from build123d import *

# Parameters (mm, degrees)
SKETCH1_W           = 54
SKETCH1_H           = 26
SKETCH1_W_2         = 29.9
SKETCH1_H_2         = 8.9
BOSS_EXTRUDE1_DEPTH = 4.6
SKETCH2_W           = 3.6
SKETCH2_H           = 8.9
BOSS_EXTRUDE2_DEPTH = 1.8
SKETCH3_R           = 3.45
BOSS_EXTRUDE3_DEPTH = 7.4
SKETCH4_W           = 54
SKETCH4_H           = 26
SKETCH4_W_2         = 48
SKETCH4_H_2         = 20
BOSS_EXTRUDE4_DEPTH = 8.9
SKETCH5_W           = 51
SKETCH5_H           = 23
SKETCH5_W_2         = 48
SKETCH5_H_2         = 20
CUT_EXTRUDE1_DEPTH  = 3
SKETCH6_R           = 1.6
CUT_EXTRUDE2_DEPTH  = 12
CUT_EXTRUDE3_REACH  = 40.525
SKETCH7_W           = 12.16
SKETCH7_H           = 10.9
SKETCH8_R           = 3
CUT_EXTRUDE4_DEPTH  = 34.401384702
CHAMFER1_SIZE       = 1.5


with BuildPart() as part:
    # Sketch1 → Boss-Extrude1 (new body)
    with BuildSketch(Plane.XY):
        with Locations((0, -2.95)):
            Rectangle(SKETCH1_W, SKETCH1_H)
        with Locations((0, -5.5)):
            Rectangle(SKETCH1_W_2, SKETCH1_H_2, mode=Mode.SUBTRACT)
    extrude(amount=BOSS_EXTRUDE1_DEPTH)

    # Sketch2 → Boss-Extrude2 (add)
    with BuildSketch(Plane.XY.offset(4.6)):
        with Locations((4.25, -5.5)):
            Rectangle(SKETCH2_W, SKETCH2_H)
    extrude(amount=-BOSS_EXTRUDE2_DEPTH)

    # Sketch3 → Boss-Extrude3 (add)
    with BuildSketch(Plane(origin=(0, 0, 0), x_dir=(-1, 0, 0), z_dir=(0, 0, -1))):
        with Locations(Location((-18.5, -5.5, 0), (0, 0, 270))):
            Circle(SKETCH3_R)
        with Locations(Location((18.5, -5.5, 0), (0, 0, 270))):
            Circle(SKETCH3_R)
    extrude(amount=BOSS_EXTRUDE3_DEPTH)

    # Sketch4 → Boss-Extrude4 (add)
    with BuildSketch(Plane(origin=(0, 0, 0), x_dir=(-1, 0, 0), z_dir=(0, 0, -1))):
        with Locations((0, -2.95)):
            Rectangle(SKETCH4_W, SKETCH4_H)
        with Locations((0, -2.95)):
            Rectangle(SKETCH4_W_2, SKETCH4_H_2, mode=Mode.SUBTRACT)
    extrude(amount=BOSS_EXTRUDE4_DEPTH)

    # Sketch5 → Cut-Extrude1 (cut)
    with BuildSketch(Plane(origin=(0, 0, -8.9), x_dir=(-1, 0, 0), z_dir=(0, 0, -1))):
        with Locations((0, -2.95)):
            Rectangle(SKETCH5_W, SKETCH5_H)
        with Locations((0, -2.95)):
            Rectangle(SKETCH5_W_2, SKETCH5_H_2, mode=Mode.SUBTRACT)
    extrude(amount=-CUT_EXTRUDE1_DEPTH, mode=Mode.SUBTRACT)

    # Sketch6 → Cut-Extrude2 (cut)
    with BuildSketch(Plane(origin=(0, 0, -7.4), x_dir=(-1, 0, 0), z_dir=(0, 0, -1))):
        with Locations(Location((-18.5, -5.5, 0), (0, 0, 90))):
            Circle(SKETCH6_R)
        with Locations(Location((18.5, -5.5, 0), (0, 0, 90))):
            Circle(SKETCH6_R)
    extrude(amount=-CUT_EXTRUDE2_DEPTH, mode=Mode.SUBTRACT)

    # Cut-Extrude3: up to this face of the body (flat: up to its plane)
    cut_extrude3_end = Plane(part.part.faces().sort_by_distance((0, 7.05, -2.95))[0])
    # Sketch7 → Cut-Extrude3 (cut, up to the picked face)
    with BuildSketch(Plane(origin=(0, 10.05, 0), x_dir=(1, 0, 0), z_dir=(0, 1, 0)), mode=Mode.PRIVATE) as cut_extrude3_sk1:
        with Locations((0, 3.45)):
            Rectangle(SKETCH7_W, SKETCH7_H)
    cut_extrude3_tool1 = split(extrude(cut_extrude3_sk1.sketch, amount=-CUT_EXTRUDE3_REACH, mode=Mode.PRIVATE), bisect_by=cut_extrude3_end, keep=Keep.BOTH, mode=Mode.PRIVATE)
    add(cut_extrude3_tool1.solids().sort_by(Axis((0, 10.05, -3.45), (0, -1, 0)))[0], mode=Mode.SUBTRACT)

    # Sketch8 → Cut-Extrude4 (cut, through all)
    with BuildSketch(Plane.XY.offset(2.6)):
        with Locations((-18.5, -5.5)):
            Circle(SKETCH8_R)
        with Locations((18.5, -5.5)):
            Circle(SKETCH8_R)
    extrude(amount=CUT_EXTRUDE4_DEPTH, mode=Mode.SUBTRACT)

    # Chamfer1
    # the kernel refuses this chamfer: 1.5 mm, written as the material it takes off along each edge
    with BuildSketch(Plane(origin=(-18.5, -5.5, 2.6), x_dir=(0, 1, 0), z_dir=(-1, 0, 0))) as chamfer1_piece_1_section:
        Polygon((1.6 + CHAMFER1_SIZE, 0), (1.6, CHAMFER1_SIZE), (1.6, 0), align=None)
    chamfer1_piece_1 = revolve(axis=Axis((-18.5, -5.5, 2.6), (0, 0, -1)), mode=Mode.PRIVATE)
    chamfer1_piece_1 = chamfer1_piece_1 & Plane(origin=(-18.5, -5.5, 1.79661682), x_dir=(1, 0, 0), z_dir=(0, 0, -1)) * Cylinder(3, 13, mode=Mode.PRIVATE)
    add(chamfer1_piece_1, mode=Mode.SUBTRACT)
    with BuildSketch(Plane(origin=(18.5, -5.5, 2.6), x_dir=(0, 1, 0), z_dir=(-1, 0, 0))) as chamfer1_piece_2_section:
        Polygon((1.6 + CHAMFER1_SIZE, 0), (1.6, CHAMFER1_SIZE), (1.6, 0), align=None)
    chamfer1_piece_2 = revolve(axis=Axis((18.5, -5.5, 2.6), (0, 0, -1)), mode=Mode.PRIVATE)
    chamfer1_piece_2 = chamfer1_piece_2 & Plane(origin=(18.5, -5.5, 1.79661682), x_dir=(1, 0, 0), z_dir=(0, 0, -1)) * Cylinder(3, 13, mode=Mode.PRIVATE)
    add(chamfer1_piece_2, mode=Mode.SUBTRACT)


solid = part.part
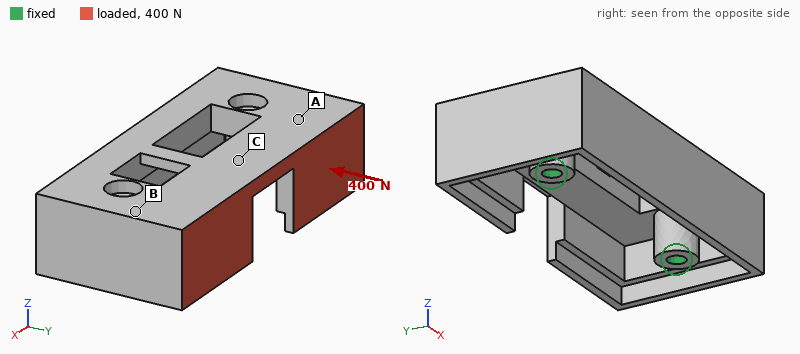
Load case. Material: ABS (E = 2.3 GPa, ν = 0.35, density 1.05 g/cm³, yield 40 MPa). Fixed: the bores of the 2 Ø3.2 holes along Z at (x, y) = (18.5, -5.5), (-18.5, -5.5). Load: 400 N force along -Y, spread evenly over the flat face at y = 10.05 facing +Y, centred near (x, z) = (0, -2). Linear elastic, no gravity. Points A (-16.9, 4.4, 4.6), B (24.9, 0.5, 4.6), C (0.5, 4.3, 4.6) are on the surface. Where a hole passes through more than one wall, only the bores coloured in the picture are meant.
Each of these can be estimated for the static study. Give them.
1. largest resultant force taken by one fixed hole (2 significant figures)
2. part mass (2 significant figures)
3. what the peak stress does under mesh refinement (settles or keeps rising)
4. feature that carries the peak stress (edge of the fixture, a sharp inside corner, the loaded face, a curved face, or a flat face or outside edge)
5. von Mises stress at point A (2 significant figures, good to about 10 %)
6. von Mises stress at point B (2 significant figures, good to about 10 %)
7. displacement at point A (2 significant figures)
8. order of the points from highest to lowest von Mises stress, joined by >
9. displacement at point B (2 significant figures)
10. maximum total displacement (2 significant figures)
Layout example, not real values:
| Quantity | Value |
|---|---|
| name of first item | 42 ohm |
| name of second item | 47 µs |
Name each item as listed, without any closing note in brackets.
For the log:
| Quantity | Value |
|---|---|
| largest resultant force taken by one fixed hole | 200 N |
| part mass | 8.9 g |
| what the peak stress does under mesh refinement | keeps rising |
| feature that carries the peak stress | a sharp inside corner |
| von Mises stress at point A | 4.3 MPa |
| von Mises stress at point B | 5.8 MPa |
| displacement at point A | 0.13 mm |
| order of the points from highest to lowest von Mises stress, joined by > | B > A > C |
| displacement at point B | 0.098 mm |
| maximum total displacement | 0.62 mm |
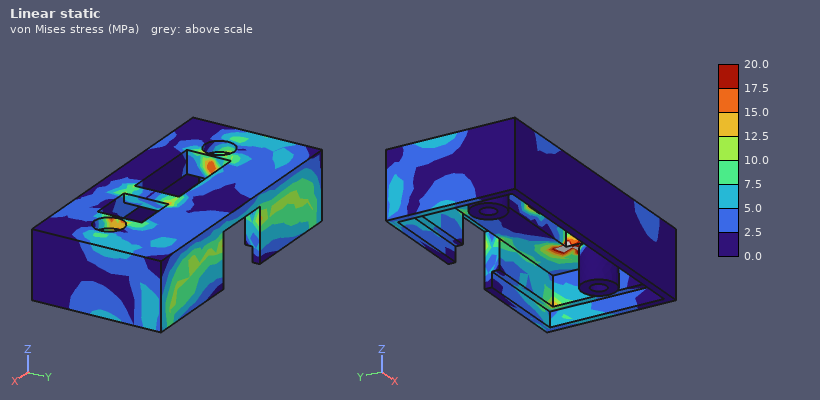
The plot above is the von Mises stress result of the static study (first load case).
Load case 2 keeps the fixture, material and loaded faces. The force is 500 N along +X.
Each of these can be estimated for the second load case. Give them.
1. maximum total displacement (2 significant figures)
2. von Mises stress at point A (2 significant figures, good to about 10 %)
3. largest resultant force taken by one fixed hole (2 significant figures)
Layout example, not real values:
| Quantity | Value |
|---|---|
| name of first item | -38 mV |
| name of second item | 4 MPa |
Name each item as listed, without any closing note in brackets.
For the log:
| Quantity | Value |
|---|---|
| maximum total displacement | 0.44 mm |
| von Mises stress at point A | 4.4 MPa |
| largest resultant force taken by one fixed hole | 300 N |
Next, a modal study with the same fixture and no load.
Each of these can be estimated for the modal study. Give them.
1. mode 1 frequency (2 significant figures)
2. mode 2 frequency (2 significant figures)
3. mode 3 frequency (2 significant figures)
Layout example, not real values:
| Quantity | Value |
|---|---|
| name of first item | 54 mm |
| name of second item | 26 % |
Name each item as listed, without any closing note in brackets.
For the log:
| Quantity | Value |
|---|---|
| mode 1 frequency | 1600 Hz |
| mode 2 frequency | 2300 Hz |
| mode 3 frequency | 2600 Hz |
